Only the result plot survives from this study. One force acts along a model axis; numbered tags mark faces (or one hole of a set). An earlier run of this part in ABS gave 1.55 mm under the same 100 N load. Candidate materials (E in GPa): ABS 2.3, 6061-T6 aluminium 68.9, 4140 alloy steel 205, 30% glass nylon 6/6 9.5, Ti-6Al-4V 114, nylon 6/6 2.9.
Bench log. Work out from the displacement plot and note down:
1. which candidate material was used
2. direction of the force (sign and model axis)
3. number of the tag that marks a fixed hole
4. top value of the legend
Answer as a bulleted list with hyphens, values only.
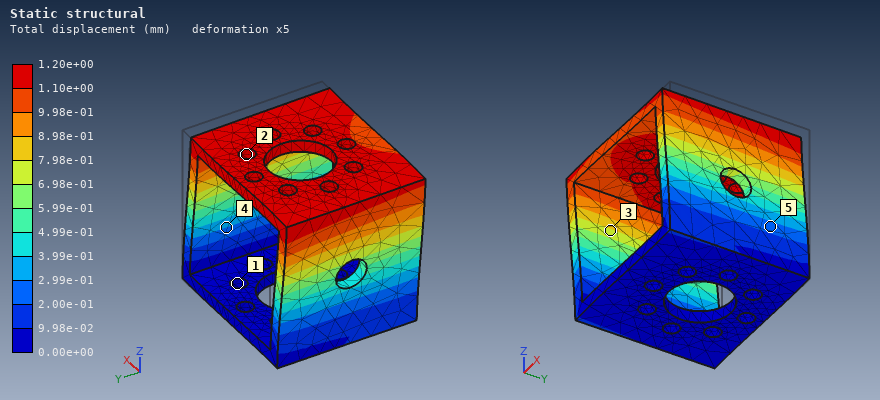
- nylon 6/6
- -X
- 1
- 1.20e+00 mm
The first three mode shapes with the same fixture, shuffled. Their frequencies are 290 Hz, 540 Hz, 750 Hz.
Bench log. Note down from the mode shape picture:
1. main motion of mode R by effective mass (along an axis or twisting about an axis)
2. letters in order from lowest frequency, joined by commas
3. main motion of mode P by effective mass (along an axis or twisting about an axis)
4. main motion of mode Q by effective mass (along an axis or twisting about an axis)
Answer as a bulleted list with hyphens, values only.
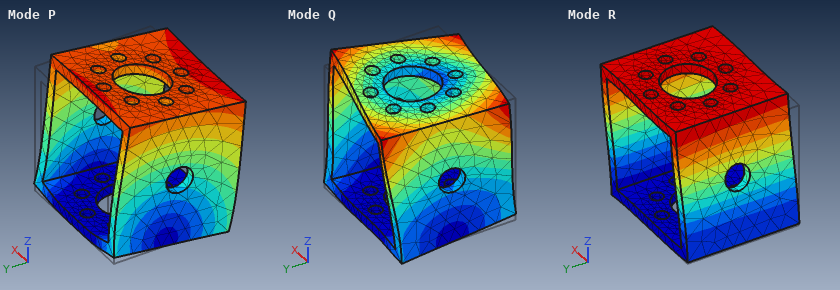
- along X
- R, P, Q
- along Y
- twisting about Z
